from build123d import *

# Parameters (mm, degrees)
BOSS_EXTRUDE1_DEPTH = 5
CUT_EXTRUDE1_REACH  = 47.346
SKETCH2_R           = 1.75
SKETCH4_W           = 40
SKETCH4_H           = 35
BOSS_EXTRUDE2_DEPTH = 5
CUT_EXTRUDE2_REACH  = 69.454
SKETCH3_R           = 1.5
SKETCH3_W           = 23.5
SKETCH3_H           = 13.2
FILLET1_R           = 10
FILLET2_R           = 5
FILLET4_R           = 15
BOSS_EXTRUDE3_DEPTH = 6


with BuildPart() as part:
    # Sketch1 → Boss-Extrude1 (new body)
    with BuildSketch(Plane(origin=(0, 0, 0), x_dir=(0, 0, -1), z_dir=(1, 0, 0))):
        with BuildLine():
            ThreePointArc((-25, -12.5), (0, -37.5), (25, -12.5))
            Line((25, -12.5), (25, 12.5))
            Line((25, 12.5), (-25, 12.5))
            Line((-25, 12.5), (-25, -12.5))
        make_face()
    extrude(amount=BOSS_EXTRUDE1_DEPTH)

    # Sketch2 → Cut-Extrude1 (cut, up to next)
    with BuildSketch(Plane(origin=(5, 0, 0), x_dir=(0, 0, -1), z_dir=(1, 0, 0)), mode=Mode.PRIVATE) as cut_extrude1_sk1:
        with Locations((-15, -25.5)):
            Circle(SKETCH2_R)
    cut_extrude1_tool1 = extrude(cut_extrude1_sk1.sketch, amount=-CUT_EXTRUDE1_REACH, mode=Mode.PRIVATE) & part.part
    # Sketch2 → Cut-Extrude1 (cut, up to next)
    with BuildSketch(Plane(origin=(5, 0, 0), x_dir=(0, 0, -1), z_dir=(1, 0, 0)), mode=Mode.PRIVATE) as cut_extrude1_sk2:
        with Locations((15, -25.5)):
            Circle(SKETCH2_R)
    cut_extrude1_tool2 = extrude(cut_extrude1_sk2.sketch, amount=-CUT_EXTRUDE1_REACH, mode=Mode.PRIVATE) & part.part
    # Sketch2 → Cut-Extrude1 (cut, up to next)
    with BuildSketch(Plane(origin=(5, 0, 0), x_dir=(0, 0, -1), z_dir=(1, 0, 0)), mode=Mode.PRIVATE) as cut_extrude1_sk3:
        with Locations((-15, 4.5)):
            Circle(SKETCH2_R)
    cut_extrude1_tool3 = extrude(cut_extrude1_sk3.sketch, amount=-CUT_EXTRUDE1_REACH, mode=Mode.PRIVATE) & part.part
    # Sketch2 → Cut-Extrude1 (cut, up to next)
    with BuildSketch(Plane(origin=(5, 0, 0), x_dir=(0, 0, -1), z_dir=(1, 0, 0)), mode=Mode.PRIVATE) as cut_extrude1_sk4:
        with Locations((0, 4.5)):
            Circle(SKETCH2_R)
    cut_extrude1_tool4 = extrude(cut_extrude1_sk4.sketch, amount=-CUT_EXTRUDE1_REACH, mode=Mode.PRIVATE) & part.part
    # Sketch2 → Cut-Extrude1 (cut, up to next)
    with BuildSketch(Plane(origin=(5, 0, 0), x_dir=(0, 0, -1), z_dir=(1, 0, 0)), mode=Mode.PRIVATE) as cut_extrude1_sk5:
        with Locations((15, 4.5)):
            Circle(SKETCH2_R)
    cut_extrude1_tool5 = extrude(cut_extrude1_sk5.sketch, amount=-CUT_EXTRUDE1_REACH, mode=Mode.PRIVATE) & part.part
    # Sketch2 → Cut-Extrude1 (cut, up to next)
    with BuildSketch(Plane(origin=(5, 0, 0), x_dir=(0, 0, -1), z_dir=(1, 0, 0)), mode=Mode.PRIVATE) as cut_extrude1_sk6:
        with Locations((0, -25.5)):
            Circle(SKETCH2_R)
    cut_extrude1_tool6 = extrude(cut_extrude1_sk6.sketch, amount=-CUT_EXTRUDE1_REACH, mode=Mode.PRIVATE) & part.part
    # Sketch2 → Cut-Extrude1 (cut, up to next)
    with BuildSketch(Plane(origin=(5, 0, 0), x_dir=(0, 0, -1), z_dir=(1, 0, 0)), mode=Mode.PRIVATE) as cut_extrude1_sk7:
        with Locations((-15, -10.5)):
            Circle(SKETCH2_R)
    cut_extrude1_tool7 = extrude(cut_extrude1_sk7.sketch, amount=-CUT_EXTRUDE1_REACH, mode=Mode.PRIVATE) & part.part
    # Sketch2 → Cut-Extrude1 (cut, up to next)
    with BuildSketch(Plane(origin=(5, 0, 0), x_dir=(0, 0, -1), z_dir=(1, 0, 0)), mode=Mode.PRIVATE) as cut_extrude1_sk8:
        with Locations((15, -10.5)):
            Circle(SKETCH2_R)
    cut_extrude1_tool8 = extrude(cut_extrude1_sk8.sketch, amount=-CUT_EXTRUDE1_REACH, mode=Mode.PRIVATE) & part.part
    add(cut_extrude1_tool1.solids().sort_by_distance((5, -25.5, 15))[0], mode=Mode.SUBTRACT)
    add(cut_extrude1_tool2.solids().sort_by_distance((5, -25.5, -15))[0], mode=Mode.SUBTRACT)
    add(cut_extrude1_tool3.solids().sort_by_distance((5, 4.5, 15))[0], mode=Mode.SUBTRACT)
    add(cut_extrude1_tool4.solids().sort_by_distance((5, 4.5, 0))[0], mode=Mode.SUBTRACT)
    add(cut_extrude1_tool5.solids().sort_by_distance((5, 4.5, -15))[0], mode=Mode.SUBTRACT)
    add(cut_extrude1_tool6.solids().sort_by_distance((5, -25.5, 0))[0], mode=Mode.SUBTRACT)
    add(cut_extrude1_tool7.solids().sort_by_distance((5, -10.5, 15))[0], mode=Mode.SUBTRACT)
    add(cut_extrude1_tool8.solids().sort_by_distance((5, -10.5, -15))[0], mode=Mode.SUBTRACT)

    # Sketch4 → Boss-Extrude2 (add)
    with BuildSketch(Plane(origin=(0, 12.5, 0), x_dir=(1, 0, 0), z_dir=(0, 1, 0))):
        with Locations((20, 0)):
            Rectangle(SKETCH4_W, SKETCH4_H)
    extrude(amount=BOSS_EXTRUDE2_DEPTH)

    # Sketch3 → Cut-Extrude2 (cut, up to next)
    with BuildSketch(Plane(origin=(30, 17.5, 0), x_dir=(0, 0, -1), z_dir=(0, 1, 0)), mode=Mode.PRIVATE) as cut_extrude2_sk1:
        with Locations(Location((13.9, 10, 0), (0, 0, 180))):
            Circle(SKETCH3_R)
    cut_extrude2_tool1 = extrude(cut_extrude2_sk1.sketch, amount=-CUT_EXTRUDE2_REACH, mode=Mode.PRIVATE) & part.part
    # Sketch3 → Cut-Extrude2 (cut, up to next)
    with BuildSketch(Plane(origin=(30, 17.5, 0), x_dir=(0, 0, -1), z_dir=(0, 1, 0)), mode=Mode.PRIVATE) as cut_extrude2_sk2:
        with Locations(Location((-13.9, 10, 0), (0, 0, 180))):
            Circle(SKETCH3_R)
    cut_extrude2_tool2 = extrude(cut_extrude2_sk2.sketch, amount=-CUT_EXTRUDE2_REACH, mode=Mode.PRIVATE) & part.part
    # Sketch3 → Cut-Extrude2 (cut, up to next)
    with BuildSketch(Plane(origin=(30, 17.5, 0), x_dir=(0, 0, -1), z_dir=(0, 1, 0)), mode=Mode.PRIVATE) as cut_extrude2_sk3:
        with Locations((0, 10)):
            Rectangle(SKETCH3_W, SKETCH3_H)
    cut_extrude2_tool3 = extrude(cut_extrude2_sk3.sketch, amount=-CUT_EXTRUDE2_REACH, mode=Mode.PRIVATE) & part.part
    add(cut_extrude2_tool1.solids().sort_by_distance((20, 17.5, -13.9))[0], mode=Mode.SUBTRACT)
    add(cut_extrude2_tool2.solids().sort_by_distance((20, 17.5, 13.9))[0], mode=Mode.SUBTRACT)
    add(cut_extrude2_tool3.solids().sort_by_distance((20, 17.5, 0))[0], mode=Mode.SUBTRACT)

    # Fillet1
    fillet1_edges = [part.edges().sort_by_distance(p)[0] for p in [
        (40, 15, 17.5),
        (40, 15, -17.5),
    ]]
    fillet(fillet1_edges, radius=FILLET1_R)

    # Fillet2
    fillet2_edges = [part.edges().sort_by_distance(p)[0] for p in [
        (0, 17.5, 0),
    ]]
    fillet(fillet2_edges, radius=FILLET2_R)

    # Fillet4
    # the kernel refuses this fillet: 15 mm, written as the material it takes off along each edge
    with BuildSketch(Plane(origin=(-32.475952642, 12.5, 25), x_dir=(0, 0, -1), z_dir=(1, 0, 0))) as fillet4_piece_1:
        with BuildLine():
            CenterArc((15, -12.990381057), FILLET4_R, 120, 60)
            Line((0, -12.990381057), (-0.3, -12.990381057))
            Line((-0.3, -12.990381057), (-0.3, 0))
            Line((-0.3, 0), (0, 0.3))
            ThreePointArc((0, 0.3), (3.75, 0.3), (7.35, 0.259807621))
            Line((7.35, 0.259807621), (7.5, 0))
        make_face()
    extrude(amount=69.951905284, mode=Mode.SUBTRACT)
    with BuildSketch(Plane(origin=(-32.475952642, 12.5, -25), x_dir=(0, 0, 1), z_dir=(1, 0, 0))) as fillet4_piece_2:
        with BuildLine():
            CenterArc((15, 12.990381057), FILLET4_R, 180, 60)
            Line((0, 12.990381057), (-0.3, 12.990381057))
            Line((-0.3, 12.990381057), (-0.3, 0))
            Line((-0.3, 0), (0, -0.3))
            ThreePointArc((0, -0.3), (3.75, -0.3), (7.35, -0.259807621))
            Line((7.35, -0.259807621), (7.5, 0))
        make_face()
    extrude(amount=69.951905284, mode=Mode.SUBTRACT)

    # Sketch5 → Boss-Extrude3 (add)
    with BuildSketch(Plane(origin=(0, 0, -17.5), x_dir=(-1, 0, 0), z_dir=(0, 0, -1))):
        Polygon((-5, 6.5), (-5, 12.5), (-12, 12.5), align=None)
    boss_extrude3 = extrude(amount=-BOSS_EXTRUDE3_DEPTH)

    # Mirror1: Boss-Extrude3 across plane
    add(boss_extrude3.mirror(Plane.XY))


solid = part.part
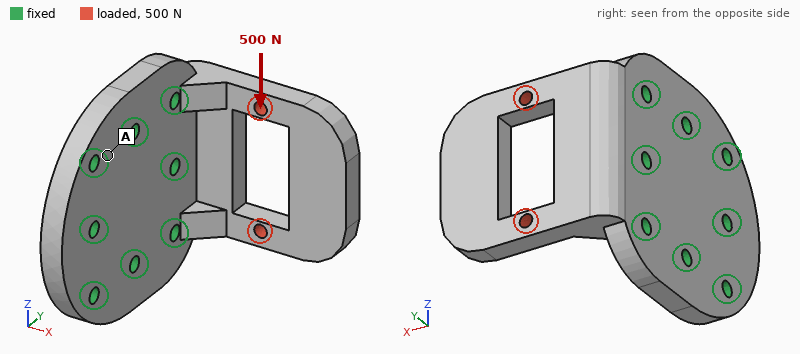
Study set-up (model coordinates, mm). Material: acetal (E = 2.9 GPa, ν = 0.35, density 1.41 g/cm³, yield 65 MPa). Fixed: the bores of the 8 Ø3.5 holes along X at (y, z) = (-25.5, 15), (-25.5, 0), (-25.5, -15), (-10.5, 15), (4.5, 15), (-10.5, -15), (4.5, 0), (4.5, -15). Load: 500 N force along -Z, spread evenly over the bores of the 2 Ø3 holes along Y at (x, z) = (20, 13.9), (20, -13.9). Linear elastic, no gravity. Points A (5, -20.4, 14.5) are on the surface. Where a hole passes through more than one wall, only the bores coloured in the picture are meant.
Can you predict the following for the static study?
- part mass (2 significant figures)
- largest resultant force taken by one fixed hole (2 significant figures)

22 g
350 N
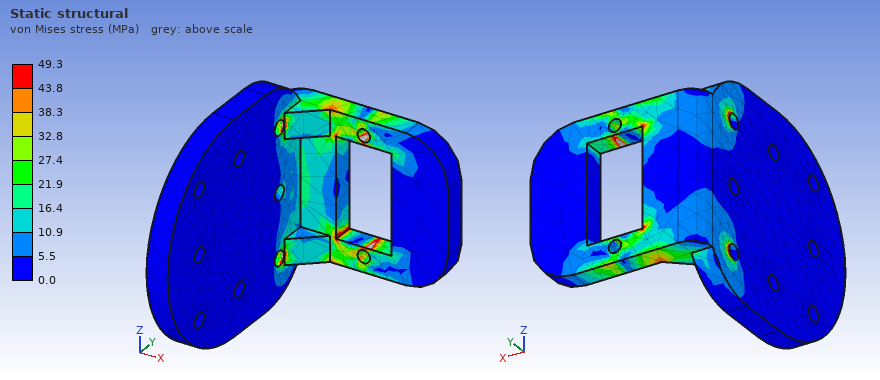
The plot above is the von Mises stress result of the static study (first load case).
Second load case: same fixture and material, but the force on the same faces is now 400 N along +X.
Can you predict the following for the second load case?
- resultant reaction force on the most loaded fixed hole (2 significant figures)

160 N
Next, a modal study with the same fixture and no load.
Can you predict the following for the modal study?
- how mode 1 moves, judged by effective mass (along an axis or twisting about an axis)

along Y
